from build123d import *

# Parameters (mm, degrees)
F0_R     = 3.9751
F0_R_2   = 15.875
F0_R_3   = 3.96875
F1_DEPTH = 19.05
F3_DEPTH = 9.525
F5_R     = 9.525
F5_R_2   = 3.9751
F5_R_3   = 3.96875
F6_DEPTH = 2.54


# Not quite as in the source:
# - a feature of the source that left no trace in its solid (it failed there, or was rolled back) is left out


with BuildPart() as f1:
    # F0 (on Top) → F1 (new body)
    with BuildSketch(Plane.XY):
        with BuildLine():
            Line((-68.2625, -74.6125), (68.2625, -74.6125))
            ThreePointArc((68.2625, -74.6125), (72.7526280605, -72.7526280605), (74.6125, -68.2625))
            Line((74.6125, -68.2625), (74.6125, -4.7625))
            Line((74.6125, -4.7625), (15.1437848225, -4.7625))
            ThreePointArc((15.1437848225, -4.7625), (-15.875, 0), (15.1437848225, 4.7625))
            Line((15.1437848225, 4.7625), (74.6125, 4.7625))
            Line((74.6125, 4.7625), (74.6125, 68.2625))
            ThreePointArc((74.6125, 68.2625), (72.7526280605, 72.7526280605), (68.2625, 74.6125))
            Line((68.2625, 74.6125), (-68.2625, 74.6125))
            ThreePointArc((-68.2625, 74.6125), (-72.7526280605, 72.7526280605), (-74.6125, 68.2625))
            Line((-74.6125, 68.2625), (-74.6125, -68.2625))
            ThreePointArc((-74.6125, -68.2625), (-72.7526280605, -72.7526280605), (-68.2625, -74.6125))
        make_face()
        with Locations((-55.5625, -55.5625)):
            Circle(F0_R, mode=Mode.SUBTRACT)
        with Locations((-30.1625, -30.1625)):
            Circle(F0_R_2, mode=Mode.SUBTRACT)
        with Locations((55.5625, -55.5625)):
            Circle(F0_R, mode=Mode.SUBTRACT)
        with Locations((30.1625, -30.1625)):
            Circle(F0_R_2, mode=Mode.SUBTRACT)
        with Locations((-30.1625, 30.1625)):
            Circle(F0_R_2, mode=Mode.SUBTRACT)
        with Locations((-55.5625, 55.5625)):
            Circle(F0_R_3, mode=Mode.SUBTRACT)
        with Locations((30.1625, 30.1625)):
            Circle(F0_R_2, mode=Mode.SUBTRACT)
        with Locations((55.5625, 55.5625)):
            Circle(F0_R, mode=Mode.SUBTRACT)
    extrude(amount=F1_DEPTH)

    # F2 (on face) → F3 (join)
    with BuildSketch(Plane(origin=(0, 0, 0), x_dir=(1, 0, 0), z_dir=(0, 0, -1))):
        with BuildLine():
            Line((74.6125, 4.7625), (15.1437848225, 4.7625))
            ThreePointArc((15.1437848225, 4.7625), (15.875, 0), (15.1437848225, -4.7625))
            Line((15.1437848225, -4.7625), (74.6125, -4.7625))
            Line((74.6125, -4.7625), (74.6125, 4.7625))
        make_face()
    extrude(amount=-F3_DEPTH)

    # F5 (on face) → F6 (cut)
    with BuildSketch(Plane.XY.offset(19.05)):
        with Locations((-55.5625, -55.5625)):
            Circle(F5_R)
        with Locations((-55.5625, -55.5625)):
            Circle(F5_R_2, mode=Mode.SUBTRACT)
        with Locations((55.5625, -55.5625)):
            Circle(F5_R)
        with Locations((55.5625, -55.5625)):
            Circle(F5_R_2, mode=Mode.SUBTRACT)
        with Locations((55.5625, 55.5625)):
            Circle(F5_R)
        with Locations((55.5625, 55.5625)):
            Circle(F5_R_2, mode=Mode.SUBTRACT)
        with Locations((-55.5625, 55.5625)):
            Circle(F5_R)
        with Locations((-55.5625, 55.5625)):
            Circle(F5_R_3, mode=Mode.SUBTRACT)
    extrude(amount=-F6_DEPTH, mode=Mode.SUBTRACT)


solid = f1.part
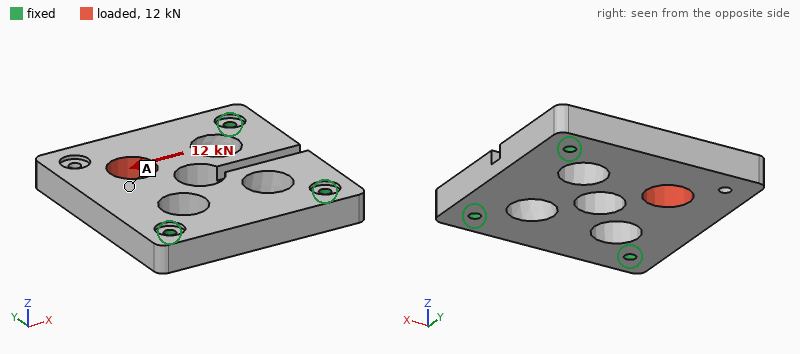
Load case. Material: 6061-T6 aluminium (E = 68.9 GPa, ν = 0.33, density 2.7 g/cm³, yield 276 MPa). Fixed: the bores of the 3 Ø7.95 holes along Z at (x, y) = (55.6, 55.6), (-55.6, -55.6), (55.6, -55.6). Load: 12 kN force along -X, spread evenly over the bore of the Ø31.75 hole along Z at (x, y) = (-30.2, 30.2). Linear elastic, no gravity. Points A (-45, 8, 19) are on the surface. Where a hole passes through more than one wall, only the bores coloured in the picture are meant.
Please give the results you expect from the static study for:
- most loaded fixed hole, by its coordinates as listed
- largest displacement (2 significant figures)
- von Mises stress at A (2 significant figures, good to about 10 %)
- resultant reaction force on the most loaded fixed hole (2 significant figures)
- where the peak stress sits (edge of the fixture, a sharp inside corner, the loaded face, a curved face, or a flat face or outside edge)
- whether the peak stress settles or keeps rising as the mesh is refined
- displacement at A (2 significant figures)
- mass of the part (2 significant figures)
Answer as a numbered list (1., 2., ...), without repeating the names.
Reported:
1. (55.6, 55.6)
2. 22 µm
3. 5.9 MPa
4. 7.7 kN
5. edge of the fixture
6. keeps rising
7. 18 µm
8. 910 g
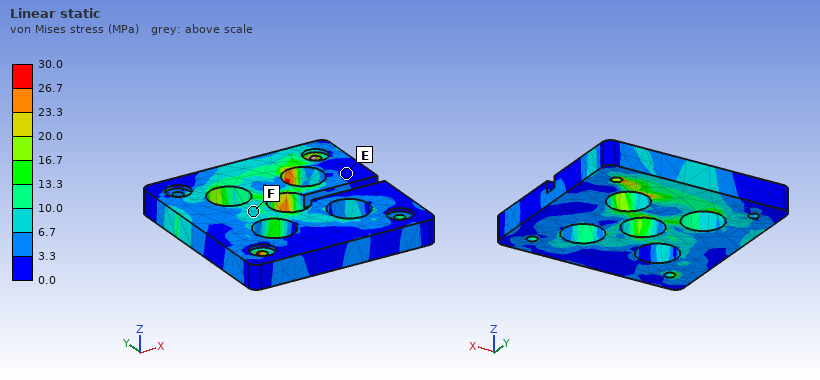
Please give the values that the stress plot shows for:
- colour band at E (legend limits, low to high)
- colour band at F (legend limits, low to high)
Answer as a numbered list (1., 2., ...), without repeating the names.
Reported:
1. 0.0 to 3.3 MPa
2. 6.7 to 10.0 MPa
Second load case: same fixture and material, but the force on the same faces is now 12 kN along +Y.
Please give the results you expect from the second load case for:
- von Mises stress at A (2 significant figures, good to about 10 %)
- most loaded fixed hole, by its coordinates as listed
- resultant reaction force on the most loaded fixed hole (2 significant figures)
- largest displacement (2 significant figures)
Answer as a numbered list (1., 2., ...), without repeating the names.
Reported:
1. 10 MPa
2. (-55.6, -55.6)
3. 7.7 kN
4. 23 µm
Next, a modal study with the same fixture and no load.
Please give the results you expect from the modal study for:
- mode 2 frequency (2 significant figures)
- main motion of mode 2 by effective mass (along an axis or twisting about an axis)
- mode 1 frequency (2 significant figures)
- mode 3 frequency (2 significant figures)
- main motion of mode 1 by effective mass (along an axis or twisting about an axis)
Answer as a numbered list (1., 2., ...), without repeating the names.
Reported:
1. 4000 Hz
2. along Z
3. 1400 Hz
4. 4700 Hz
5. along Z
